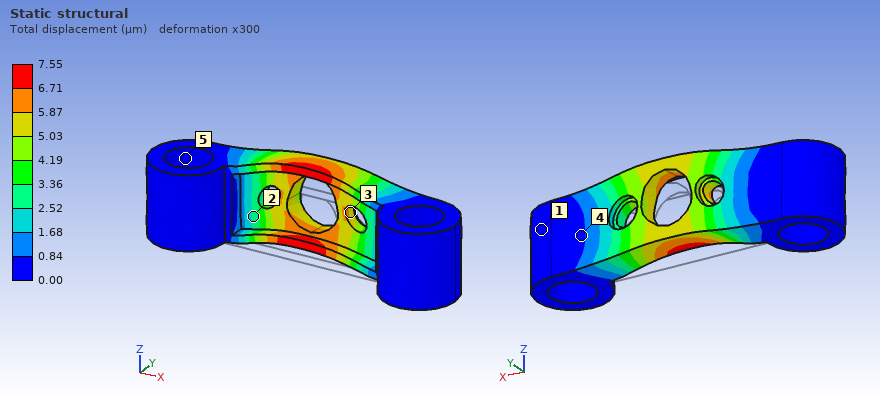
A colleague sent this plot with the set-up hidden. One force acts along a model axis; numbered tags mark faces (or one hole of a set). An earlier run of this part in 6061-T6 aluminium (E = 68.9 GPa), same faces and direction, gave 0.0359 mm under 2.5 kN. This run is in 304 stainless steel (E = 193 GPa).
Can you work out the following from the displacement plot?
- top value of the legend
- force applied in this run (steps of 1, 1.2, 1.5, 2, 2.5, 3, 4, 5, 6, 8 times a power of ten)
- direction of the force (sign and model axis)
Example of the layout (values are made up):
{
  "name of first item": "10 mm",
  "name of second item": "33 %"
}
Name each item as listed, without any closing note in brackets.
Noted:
{
  "top value of the legend": "7.55 µm",
  "force applied in this run": "1.5 kN",
  "direction of the force": "+Z"
}
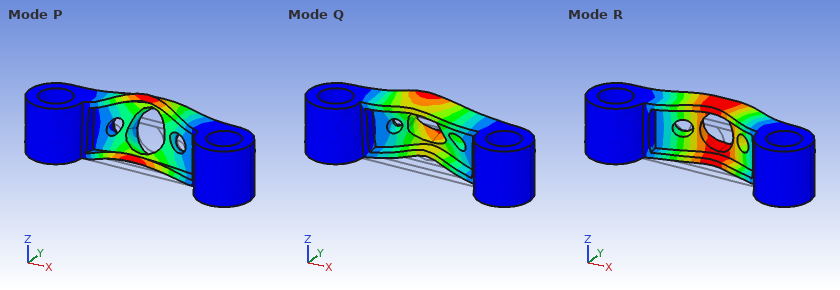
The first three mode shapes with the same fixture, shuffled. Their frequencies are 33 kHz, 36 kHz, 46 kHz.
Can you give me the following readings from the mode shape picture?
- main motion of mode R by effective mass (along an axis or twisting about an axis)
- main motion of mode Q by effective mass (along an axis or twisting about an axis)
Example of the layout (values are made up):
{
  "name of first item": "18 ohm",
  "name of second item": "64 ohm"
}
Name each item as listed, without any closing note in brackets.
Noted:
{
  "main motion of mode R by effective mass": "along Y",
  "main motion of mode Q by effective mass": "along Z"
}
